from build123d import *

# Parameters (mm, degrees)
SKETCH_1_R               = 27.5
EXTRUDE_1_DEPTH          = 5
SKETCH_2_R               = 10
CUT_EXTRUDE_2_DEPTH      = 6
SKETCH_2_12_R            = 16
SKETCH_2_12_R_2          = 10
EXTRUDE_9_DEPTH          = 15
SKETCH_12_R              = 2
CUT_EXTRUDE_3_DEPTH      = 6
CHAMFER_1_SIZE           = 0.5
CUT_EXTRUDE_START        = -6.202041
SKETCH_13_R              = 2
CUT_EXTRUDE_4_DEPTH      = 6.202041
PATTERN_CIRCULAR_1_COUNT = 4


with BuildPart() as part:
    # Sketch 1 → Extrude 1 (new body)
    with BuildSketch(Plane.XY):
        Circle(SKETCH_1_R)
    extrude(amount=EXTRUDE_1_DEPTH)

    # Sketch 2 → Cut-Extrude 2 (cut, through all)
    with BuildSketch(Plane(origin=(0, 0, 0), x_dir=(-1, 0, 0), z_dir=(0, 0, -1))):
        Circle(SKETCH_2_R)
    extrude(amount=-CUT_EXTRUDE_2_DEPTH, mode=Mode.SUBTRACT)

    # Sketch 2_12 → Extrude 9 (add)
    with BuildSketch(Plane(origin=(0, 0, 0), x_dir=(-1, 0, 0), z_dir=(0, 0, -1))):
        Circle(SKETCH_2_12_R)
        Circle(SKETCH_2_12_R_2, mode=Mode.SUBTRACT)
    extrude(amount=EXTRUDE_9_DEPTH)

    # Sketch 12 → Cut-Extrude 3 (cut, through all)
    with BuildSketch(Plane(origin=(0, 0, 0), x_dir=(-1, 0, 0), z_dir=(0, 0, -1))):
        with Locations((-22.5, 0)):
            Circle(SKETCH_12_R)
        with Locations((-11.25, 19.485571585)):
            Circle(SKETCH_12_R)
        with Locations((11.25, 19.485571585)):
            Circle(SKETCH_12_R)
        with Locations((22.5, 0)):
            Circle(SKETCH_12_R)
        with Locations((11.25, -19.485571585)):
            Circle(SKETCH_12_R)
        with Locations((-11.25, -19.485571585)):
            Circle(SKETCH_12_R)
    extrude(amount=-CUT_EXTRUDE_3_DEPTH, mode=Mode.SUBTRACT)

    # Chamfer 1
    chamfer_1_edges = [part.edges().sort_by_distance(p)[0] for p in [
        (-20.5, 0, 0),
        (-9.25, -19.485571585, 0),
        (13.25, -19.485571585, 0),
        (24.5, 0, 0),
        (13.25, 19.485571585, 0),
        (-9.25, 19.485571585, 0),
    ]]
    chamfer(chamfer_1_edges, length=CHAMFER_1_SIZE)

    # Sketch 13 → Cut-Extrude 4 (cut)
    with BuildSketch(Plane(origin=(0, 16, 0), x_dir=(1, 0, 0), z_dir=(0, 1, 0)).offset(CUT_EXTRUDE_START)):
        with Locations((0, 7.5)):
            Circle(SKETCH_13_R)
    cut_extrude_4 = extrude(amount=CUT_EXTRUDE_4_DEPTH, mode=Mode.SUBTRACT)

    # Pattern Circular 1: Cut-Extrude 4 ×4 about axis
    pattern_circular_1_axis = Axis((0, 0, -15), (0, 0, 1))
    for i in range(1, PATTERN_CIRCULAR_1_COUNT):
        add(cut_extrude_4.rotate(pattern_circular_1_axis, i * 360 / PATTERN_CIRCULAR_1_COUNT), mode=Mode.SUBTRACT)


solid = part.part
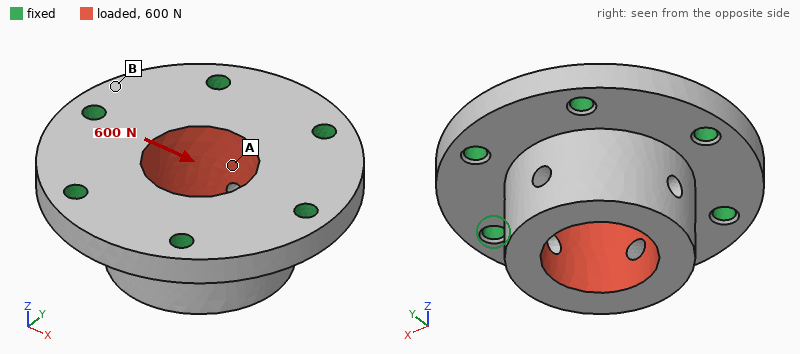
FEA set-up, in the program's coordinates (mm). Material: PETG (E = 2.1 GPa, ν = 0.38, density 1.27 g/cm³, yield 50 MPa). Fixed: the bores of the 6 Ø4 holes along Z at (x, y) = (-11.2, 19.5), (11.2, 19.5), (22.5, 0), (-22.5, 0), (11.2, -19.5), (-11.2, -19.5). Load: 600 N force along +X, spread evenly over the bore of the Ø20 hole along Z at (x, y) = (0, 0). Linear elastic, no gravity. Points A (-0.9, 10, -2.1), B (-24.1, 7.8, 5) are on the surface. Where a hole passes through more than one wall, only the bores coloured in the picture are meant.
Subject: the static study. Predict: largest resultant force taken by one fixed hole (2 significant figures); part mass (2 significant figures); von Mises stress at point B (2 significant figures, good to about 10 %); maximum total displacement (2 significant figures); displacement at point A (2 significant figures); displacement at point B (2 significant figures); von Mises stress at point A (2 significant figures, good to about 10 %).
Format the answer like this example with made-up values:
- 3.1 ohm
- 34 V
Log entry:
- 160 N
- 22 g
- 0.99 MPa
- 55 µm
- 18 µm
- 8.5 µm
- 2.5 MPa
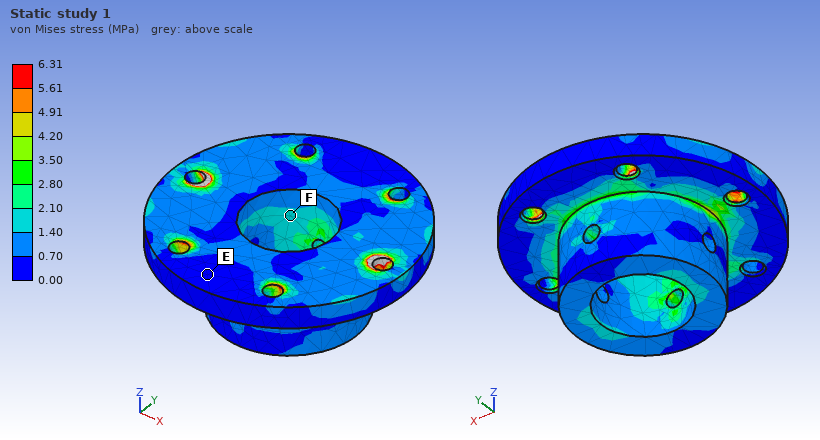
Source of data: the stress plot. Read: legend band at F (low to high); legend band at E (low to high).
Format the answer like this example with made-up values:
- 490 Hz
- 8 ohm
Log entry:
- 1.40 to 2.10 MPa
- 0.00 to 0.70 MPa
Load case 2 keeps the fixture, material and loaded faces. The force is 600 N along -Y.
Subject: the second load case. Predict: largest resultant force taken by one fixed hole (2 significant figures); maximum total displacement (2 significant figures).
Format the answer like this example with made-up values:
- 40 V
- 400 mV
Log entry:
- 140 N
- 54 µm
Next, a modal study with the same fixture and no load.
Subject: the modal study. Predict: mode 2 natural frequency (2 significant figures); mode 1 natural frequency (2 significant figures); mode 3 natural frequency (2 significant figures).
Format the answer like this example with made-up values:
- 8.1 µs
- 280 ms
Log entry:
- 5400 Hz
- 5400 Hz
- 5500 Hz
